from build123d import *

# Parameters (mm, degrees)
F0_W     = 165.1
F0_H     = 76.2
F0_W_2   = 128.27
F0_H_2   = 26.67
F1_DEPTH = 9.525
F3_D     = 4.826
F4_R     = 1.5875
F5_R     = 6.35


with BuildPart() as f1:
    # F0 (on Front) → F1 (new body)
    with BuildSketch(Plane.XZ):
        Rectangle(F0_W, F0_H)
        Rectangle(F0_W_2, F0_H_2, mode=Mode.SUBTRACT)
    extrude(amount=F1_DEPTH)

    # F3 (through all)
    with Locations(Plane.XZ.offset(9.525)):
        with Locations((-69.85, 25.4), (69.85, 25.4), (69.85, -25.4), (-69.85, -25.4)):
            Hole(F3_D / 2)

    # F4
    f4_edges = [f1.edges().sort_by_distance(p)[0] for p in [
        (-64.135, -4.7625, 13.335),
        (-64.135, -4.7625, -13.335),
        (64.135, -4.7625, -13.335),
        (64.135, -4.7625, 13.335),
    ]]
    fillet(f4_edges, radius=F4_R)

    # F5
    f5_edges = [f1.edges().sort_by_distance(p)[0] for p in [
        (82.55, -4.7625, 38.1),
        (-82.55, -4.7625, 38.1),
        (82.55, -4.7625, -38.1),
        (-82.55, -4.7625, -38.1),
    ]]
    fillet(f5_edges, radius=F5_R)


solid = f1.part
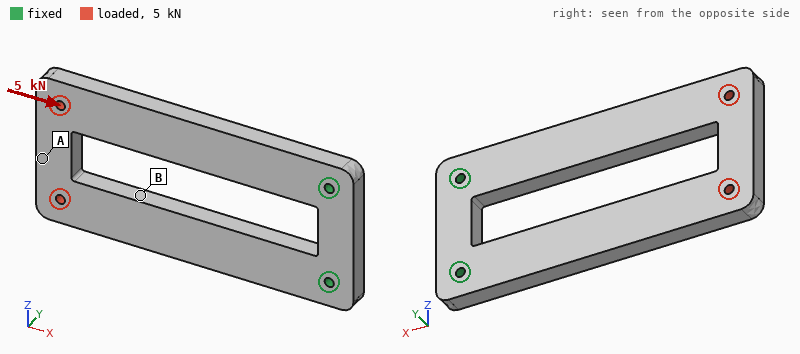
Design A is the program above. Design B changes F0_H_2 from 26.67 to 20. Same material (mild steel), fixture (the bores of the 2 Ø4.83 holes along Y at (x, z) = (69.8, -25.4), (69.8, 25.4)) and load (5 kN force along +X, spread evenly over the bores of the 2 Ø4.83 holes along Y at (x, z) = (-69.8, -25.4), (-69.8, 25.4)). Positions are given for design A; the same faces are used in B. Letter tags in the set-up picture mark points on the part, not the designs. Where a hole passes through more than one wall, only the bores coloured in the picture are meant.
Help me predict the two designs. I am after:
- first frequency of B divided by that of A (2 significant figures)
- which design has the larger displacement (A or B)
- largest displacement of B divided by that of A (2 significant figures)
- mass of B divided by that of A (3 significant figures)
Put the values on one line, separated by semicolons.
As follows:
1.0; A; 0.91; 1.09
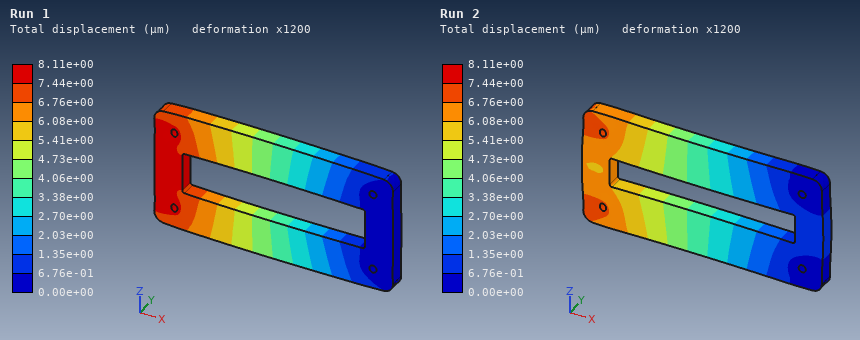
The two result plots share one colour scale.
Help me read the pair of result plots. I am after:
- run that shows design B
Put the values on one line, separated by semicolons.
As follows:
Run 2
